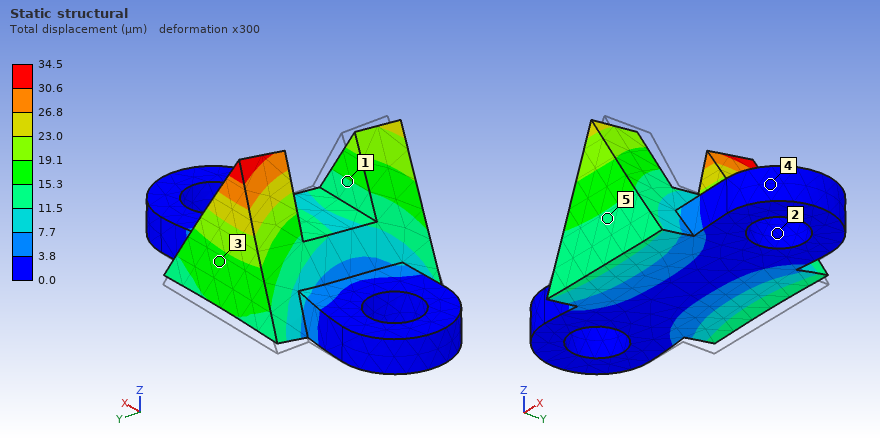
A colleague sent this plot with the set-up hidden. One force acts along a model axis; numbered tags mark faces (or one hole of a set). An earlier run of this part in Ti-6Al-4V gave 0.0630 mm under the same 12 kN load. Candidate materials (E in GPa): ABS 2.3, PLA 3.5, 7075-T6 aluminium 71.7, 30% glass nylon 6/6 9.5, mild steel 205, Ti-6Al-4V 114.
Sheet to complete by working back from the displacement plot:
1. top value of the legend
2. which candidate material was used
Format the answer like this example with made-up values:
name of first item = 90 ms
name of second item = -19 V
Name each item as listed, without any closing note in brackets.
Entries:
top value of the legend = 34.5 µm
which candidate material was used = mild steel
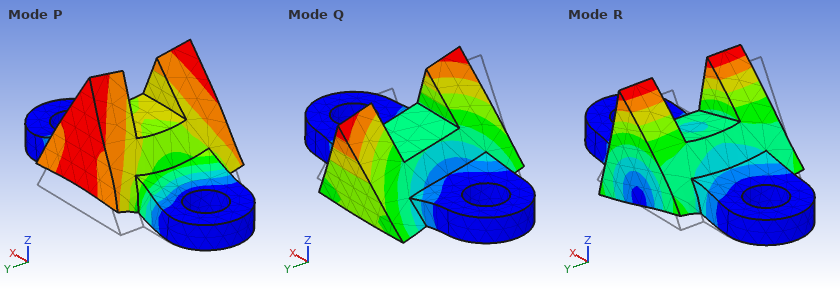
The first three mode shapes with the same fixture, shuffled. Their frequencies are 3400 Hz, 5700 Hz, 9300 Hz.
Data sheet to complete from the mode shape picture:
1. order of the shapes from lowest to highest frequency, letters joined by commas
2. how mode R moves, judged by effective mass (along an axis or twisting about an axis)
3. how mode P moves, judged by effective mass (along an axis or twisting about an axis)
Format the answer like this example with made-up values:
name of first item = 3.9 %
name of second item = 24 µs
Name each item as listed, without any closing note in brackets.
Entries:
order of the shapes from lowest to highest frequency, letters joined by commas = Q, P, R
how mode R moves, judged by effective mass = along X
how mode P moves, judged by effective mass = along Z
